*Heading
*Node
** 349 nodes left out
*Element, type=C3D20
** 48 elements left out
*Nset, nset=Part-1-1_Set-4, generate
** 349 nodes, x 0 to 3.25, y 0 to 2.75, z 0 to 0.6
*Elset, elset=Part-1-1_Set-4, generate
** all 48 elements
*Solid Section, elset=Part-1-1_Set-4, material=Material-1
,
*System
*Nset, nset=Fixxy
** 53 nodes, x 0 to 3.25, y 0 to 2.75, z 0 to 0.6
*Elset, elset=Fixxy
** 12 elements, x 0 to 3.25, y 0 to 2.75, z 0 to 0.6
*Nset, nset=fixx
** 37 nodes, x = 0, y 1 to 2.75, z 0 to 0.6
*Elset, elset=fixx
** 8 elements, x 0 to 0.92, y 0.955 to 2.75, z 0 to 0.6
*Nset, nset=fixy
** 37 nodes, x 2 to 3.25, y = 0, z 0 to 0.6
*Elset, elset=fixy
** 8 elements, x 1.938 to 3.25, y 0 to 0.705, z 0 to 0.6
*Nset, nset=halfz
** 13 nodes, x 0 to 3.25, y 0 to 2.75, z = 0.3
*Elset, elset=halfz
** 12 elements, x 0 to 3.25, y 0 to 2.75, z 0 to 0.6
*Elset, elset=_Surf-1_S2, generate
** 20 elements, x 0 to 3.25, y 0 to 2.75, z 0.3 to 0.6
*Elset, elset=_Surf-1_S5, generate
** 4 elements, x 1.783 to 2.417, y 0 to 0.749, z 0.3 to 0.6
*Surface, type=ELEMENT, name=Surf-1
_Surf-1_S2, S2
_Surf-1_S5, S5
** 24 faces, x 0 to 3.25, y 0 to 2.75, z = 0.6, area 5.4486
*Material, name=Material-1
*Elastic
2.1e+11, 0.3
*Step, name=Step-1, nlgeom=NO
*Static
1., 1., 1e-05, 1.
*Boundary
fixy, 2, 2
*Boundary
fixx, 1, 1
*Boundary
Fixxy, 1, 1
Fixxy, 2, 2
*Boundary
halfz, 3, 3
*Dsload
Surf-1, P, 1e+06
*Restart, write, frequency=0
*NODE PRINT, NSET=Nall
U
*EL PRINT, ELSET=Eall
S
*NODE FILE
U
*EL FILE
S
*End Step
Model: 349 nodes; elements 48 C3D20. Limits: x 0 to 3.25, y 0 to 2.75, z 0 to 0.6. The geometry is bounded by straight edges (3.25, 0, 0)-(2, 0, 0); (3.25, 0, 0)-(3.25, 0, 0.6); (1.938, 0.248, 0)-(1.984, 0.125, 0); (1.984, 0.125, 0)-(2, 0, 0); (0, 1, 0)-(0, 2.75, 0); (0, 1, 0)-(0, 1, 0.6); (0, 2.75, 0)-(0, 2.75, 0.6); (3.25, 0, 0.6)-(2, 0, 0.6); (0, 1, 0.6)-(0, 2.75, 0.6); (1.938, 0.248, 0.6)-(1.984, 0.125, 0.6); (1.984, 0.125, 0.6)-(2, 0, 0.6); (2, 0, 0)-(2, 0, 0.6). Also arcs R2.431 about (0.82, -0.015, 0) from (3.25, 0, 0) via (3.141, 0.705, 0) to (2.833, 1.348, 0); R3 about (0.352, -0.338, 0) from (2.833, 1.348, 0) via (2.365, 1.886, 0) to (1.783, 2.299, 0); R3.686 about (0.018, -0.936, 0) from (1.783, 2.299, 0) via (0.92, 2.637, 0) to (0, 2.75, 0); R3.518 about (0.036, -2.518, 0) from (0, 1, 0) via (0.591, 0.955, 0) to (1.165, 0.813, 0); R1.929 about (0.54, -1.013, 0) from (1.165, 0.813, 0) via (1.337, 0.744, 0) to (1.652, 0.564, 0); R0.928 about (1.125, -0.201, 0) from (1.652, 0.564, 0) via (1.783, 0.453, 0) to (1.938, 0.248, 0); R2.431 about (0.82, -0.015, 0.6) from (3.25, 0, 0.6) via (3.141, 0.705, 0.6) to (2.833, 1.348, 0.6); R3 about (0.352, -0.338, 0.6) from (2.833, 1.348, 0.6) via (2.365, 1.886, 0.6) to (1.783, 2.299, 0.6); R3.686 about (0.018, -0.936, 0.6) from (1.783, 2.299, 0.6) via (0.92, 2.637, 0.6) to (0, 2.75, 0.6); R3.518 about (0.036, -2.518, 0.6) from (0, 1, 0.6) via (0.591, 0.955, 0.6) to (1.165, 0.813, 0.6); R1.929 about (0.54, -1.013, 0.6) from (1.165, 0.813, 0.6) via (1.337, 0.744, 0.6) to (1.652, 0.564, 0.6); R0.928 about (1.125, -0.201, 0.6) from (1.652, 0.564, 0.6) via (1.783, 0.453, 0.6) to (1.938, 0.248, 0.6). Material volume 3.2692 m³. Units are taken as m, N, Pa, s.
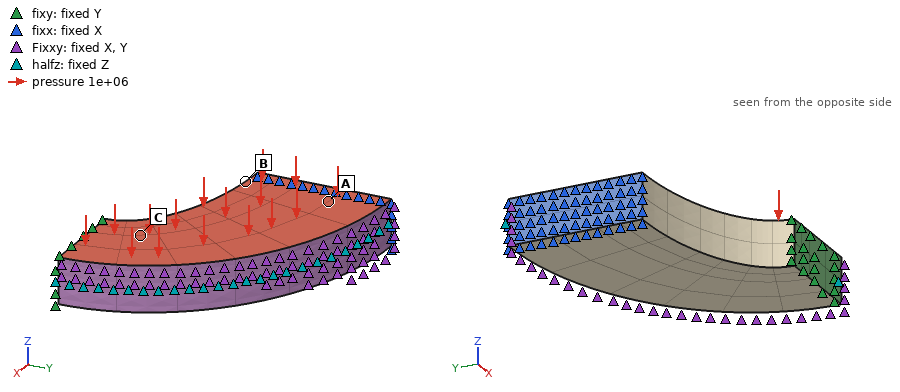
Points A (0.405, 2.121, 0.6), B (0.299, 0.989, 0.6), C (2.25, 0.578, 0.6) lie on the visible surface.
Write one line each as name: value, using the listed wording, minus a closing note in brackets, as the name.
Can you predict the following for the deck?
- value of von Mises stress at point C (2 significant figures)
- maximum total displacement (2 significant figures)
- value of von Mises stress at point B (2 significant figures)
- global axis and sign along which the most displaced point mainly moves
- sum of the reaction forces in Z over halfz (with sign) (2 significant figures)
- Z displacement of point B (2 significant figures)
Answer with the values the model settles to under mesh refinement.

value of von Mises stress at point C: 3.9e+06 Pa
maximum total displacement: 2.0e-04 m
value of von Mises stress at point B: 4.7e+06 Pa
global axis and sign along which the most displaced point mainly moves: -Z
sum of the reaction forces in Z over halfz (with sign): 5.4e+06 N
Z displacement of point B: -2.0e-04 m
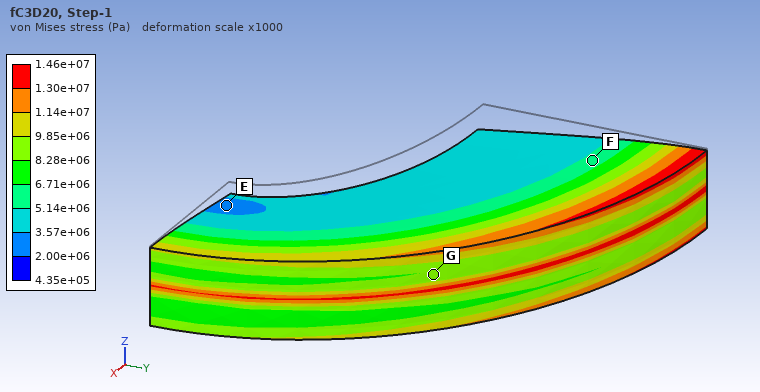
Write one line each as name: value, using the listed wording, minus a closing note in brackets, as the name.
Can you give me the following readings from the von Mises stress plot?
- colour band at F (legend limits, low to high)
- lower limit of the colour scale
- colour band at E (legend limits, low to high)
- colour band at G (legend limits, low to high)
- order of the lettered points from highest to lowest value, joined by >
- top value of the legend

colour band at F: 5.14e+06 to 6.71e+06 Pa
lower limit of the colour scale: 4.35e+05 Pa
colour band at E: 2.00e+06 to 3.57e+06 Pa
colour band at G: 8.28e+06 to 9.85e+06 Pa
order of the lettered points from highest to lowest value, joined by >: G > F > E
top value of the legend: 1.46e+07 Pa
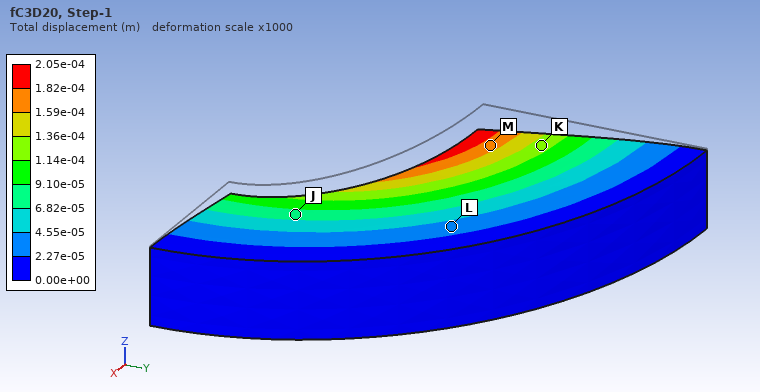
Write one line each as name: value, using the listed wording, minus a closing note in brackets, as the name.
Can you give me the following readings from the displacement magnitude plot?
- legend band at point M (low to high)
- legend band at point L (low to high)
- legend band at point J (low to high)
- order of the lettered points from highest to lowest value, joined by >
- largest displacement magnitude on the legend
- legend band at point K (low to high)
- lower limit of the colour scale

legend band at point M: 1.59e-04 to 1.82e-04 m
legend band at point L: 2.27e-05 to 4.55e-05 m
legend band at point J: 6.82e-05 to 9.10e-05 m
order of the lettered points from highest to lowest value, joined by >: M > K > J > L
largest displacement magnitude on the legend: 2.05e-04 m
legend band at point K: 1.14e-04 to 1.36e-04 m
lower limit of the colour scale: 0.00e+00 m
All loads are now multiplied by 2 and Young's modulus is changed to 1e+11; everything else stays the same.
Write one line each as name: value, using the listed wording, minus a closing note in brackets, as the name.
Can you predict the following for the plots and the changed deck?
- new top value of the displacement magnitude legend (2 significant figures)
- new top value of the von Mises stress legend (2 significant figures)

new top value of the displacement magnitude legend: 8.6e-04 m
new top value of the von Mises stress legend: 2.9e+07 Pa
